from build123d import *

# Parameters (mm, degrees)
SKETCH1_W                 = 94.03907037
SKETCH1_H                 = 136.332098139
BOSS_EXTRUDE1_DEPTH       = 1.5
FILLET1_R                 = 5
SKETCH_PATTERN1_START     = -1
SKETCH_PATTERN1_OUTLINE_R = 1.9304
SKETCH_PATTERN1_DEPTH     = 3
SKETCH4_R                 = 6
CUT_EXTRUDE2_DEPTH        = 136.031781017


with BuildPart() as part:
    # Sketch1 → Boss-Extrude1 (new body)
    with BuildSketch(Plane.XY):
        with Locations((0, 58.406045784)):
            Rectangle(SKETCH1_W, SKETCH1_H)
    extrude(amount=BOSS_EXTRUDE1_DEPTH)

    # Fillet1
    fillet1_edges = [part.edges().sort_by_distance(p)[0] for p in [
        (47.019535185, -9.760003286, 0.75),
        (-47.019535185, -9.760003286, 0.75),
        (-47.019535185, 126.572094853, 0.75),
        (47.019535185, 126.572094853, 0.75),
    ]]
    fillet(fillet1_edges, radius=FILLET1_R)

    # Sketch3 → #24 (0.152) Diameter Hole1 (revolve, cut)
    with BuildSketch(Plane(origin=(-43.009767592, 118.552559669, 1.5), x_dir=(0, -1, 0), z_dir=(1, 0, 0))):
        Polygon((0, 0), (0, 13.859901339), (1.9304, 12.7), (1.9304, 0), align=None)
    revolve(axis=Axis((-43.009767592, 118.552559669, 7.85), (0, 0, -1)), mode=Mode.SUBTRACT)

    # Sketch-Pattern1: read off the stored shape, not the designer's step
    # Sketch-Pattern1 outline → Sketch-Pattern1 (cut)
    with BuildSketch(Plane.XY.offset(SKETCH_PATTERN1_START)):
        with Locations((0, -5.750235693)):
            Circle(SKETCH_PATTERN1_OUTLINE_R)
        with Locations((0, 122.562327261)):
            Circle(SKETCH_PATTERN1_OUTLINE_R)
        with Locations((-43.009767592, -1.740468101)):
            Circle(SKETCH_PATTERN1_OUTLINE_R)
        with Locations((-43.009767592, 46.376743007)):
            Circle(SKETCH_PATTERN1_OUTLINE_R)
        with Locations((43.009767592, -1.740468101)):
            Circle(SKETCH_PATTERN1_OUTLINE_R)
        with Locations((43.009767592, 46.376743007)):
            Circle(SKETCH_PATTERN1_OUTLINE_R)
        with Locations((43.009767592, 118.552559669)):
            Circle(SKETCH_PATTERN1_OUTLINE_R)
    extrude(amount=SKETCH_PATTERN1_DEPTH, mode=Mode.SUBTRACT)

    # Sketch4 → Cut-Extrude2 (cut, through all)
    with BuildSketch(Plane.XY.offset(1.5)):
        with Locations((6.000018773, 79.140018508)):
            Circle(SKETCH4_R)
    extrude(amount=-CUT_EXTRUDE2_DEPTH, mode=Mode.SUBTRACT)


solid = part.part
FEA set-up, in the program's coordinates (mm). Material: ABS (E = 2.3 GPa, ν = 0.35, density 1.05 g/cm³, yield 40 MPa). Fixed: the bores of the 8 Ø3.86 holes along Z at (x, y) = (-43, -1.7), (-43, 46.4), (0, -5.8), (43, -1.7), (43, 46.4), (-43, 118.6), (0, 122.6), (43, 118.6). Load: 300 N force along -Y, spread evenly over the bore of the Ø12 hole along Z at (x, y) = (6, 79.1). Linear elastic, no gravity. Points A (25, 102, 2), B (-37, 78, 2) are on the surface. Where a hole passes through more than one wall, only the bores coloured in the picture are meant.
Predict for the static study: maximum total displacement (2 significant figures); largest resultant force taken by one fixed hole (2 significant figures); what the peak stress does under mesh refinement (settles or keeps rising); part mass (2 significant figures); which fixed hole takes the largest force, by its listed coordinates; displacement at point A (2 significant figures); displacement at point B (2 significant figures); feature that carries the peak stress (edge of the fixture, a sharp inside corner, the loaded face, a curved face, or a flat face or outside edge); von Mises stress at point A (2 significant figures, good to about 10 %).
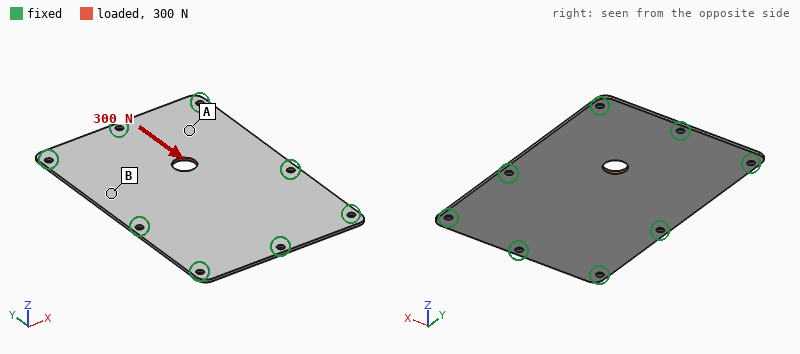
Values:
62 µm
79 N
keeps rising
20 g
(0, 122.6)
24 µm
9.8 µm
edge of the fixture
1.6 MPa
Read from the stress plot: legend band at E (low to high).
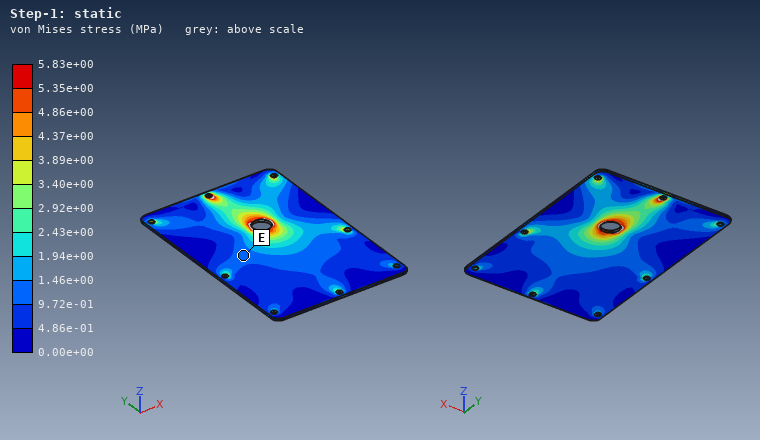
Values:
9.72e-01 to 1.46e+00 MPa
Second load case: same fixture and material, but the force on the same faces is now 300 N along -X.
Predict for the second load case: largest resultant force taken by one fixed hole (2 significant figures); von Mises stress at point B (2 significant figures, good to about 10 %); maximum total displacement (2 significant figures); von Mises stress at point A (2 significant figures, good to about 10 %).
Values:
76 N
0.64 MPa
80 µm
2.5 MPa
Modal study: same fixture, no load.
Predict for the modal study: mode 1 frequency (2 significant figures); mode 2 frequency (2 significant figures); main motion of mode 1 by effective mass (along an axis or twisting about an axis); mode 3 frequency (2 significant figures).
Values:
290 Hz
450 Hz
along Z
470 Hz
